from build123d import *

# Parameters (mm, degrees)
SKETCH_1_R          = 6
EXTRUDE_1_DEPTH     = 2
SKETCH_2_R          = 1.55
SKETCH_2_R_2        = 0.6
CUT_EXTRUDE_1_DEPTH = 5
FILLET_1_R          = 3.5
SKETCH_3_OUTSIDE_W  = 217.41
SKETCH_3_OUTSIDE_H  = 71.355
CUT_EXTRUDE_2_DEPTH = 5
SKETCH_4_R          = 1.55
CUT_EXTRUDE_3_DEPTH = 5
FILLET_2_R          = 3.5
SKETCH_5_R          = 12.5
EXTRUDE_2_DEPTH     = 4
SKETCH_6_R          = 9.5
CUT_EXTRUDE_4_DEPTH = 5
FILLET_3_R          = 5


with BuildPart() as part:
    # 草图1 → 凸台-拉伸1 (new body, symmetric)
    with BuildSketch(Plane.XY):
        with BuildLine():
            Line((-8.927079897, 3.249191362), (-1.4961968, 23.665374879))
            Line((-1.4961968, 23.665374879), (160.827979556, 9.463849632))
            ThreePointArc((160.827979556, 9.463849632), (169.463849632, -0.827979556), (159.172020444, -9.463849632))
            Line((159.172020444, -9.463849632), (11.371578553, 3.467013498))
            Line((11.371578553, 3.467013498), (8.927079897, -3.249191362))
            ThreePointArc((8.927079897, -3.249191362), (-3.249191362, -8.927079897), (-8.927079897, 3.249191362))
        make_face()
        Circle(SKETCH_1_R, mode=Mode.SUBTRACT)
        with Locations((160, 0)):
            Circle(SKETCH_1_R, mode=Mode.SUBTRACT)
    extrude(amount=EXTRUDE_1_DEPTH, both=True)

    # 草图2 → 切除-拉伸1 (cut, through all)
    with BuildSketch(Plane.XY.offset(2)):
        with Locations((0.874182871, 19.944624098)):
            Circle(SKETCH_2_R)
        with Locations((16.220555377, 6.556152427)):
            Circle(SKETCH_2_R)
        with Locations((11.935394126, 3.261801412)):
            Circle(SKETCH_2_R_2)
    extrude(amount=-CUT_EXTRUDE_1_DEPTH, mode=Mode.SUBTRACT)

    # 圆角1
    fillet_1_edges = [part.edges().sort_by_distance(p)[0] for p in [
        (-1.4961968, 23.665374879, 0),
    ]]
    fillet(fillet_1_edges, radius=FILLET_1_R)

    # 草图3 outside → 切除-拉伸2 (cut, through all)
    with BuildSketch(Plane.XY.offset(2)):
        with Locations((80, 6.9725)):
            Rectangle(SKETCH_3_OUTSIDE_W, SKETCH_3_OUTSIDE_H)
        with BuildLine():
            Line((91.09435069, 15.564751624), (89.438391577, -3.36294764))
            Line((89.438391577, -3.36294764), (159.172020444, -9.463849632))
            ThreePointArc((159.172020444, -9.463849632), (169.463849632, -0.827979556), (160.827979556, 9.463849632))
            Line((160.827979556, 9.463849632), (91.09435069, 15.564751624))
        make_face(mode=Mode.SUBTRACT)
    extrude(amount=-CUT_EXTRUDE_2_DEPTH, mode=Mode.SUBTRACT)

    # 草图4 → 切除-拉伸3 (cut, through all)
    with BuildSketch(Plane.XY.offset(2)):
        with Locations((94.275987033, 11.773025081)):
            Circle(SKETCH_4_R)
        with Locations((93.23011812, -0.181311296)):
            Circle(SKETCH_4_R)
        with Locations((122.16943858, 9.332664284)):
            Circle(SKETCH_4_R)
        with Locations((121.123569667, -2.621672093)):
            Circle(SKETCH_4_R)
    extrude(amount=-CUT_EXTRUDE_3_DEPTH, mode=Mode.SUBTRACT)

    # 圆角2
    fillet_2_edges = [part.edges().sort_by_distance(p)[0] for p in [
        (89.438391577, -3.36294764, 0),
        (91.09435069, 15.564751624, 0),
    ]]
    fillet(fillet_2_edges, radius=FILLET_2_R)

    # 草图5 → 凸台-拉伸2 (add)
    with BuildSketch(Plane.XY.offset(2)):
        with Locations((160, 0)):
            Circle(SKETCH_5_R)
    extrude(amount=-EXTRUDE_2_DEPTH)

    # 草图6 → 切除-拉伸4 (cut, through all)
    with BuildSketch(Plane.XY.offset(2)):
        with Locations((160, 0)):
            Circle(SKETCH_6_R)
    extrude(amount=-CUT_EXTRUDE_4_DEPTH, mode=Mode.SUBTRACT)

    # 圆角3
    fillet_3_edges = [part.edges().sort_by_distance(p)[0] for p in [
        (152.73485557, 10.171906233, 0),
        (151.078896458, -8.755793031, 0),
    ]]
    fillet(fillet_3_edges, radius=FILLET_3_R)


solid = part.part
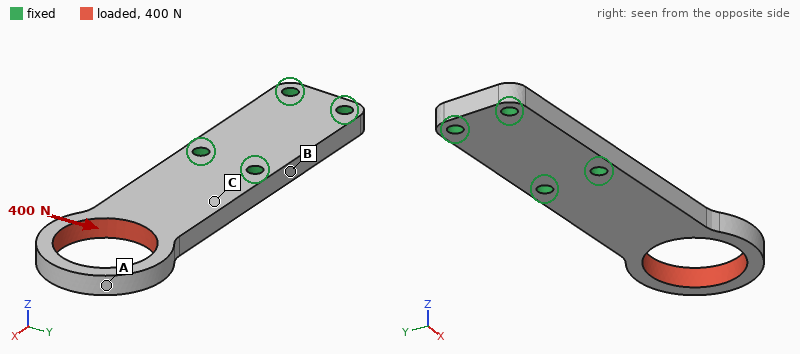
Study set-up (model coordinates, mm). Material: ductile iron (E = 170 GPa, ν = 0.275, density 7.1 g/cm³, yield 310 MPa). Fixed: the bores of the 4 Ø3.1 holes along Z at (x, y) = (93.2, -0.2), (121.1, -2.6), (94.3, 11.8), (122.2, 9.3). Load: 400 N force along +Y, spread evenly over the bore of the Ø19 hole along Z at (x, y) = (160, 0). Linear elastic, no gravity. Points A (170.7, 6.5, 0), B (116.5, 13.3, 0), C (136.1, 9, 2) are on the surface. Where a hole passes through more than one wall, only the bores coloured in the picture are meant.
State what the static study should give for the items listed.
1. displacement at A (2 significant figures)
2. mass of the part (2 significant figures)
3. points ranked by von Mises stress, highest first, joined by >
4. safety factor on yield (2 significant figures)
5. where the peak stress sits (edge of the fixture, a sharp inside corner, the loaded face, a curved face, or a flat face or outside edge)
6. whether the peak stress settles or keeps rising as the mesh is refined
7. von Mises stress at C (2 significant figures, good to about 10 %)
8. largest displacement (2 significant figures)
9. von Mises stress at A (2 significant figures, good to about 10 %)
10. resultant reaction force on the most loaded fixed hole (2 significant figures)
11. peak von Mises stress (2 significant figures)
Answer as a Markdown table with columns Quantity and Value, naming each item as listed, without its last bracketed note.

| Quantity | Value |
|---|---|
| displacement at A | 75 µm |
| mass of the part | 37 g |
| points ranked by von Mises stress, highest first, joined by > | A > C > B |
| safety factor on yield | 2.0 |
| where the peak stress sits | a curved face |
| whether the peak stress settles or keeps rising as the mesh is refined | settles |
| von Mises stress at C | 31 MPa |
| largest displacement | 76 µm |
| von Mises stress at A | 57 MPa |
| resultant reaction force on the most loaded fixed hole | 1.1 kN |
| peak von Mises stress | 160 MPa |
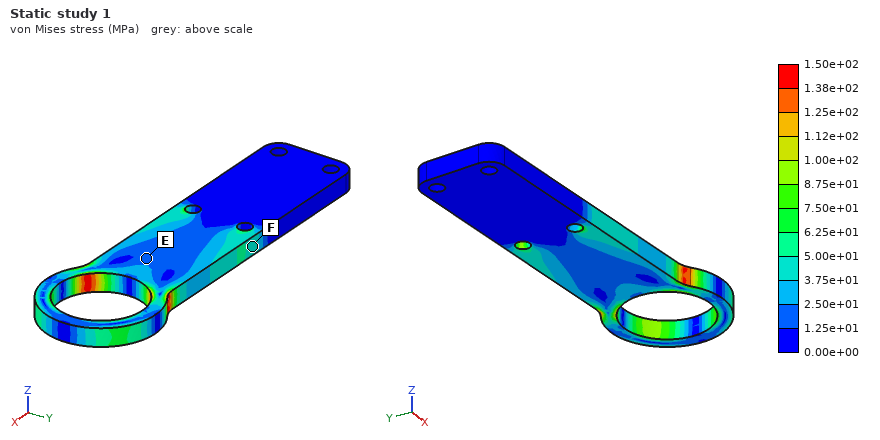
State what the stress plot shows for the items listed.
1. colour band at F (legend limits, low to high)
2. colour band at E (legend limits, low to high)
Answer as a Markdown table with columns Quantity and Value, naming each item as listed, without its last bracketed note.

| Quantity | Value |
|---|---|
| colour band at F | 3.75e+01 to 5.00e+01 MPa |
| colour band at E | 1.25e+01 to 2.50e+01 MPa |
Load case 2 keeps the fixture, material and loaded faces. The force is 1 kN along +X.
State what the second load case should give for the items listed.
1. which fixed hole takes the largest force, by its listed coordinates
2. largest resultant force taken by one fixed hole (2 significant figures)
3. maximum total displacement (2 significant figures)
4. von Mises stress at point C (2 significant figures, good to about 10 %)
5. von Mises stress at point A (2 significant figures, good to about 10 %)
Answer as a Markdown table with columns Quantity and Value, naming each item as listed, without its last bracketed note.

| Quantity | Value |
|---|---|
| which fixed hole takes the largest force, by its listed coordinates | (121.1, -2.6) |
| largest resultant force taken by one fixed hole | 730 N |
| maximum total displacement | 26 µm |
| von Mises stress at point C | 8.1 MPa |
| von Mises stress at point A | 37 MPa |
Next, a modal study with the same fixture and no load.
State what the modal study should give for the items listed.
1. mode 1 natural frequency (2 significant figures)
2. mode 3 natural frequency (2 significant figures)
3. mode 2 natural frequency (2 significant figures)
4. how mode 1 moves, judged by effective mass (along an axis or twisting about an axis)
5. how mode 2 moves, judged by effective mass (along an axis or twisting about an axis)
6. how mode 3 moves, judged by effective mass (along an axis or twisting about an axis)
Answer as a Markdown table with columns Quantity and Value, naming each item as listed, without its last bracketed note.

| Quantity | Value |
|---|---|
| mode 1 natural frequency | 1700 Hz |
| mode 3 natural frequency | 5700 Hz |
| mode 2 natural frequency | 5200 Hz |
| how mode 1 moves, judged by effective mass | along Z |
| how mode 2 moves, judged by effective mass | along Y |
| how mode 3 moves, judged by effective mass | twisting about X |
